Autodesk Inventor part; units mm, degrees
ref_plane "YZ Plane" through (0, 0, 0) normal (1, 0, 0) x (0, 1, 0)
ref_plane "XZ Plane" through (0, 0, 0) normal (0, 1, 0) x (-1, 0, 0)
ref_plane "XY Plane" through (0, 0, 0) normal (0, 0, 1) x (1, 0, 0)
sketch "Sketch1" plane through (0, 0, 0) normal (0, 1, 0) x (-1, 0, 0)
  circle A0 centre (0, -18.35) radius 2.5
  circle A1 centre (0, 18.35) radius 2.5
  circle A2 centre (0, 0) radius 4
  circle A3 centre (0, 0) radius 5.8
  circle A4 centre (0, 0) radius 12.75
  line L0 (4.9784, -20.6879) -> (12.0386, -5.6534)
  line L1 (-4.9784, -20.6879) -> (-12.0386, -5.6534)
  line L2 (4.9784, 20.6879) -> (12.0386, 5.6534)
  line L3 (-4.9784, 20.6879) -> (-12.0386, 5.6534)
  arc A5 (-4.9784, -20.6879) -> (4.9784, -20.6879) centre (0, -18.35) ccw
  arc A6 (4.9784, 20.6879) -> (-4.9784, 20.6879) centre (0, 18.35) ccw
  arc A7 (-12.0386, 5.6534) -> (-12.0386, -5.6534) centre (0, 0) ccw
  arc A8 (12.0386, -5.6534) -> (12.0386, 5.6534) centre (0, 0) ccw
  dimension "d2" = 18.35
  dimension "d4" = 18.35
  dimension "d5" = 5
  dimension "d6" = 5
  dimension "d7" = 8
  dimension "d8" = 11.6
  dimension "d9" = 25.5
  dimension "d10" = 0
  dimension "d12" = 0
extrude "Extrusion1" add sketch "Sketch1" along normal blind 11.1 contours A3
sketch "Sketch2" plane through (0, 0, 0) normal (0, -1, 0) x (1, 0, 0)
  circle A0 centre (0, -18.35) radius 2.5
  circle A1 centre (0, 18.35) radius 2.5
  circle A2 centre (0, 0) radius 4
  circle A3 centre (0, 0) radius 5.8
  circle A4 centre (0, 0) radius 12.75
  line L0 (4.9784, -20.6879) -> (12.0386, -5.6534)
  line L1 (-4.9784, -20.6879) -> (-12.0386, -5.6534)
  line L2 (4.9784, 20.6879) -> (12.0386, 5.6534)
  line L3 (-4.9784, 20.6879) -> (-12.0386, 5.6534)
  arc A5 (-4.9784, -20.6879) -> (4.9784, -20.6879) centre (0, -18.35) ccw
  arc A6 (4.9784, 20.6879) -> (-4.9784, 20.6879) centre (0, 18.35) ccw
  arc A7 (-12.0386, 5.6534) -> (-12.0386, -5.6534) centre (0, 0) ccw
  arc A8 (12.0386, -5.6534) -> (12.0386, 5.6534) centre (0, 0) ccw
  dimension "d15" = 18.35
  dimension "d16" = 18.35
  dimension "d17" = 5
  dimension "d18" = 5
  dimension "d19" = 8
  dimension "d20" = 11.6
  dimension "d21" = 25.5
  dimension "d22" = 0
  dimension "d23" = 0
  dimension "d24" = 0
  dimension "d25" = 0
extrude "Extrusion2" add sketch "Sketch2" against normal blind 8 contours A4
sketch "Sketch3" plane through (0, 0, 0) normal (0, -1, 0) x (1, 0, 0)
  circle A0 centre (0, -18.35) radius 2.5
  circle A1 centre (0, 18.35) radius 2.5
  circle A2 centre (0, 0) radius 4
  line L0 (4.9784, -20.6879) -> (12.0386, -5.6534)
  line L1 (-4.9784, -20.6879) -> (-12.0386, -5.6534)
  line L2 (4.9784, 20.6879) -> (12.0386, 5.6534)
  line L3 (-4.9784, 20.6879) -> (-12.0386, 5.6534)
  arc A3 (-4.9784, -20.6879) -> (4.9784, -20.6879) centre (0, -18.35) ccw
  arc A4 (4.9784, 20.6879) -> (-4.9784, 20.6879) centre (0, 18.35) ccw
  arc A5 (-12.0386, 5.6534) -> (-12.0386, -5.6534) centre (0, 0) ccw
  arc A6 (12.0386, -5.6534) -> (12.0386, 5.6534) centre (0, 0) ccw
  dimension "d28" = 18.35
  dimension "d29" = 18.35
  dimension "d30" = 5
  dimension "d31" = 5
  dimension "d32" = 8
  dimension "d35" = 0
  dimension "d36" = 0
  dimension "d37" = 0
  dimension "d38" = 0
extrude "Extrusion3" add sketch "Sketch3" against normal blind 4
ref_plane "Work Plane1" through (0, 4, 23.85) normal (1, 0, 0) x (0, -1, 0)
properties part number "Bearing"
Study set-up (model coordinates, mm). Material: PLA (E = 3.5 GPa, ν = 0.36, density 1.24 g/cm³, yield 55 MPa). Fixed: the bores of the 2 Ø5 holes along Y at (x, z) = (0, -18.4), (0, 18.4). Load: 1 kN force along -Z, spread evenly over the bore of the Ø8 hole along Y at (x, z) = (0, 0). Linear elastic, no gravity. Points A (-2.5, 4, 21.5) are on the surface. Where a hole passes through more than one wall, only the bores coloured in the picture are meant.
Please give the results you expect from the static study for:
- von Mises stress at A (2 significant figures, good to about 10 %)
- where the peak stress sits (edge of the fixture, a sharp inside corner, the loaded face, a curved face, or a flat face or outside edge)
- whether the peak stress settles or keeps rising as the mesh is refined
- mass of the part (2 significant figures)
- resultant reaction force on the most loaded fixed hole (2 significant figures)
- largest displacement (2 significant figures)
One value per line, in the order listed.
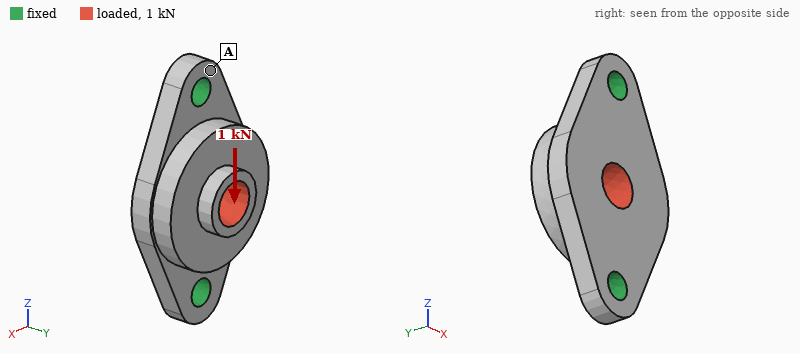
2.7 MPa
edge of the fixture
keeps rising
6.3 g
510 N
68 µm
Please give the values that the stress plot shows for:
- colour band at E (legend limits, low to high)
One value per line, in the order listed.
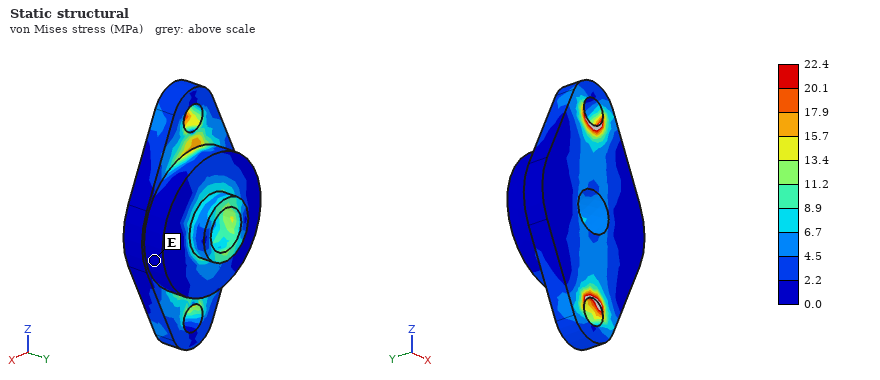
0.0 to 2.2 MPa
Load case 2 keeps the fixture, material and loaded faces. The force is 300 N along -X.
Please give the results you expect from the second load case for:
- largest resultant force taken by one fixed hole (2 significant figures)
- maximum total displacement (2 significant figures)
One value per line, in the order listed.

150 N
0.12 mm
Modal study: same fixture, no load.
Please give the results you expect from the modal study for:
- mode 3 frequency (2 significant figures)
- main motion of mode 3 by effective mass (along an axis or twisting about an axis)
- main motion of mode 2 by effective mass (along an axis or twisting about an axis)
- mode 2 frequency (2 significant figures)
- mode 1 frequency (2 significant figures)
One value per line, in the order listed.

8800 Hz
along X
along Y
5100 Hz
3500 Hz
